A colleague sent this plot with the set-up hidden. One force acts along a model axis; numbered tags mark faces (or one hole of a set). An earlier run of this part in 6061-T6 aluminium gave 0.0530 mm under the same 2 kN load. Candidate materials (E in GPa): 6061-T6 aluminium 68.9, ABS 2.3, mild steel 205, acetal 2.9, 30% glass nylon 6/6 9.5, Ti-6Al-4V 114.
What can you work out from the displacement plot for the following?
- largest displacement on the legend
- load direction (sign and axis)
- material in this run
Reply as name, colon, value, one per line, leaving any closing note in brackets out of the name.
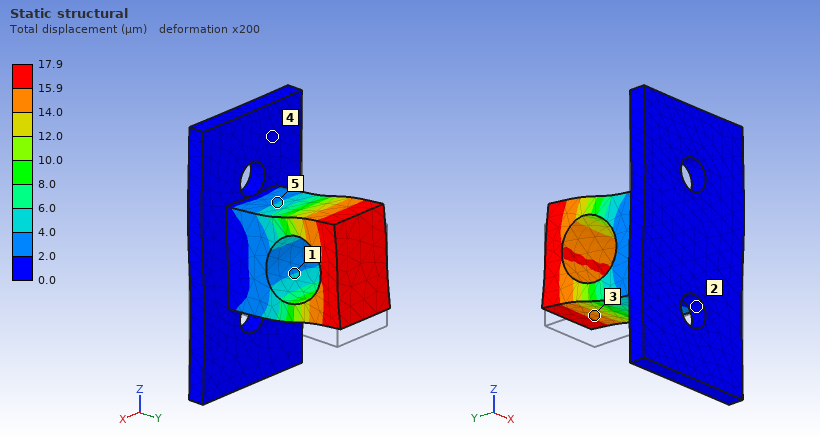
largest displacement on the legend: 17.9 µm
load direction: +Z
material in this run: mild steel
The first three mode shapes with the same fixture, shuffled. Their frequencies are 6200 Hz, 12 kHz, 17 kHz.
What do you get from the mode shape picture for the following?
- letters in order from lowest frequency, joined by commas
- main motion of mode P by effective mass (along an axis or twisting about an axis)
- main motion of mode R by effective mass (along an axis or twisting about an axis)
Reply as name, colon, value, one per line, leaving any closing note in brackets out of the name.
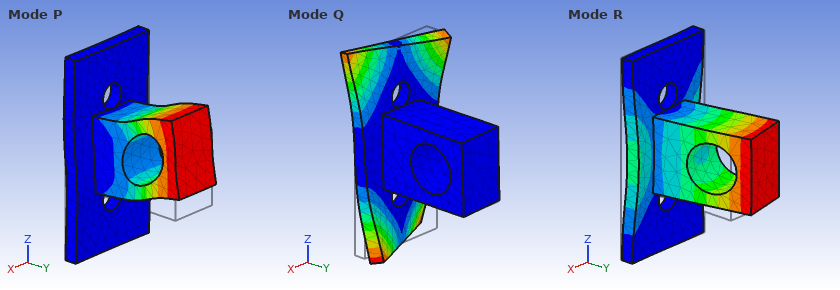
letters in order from lowest frequency, joined by commas: R, P, Q
main motion of mode P by effective mass: along Z
main motion of mode R by effective mass: along X
